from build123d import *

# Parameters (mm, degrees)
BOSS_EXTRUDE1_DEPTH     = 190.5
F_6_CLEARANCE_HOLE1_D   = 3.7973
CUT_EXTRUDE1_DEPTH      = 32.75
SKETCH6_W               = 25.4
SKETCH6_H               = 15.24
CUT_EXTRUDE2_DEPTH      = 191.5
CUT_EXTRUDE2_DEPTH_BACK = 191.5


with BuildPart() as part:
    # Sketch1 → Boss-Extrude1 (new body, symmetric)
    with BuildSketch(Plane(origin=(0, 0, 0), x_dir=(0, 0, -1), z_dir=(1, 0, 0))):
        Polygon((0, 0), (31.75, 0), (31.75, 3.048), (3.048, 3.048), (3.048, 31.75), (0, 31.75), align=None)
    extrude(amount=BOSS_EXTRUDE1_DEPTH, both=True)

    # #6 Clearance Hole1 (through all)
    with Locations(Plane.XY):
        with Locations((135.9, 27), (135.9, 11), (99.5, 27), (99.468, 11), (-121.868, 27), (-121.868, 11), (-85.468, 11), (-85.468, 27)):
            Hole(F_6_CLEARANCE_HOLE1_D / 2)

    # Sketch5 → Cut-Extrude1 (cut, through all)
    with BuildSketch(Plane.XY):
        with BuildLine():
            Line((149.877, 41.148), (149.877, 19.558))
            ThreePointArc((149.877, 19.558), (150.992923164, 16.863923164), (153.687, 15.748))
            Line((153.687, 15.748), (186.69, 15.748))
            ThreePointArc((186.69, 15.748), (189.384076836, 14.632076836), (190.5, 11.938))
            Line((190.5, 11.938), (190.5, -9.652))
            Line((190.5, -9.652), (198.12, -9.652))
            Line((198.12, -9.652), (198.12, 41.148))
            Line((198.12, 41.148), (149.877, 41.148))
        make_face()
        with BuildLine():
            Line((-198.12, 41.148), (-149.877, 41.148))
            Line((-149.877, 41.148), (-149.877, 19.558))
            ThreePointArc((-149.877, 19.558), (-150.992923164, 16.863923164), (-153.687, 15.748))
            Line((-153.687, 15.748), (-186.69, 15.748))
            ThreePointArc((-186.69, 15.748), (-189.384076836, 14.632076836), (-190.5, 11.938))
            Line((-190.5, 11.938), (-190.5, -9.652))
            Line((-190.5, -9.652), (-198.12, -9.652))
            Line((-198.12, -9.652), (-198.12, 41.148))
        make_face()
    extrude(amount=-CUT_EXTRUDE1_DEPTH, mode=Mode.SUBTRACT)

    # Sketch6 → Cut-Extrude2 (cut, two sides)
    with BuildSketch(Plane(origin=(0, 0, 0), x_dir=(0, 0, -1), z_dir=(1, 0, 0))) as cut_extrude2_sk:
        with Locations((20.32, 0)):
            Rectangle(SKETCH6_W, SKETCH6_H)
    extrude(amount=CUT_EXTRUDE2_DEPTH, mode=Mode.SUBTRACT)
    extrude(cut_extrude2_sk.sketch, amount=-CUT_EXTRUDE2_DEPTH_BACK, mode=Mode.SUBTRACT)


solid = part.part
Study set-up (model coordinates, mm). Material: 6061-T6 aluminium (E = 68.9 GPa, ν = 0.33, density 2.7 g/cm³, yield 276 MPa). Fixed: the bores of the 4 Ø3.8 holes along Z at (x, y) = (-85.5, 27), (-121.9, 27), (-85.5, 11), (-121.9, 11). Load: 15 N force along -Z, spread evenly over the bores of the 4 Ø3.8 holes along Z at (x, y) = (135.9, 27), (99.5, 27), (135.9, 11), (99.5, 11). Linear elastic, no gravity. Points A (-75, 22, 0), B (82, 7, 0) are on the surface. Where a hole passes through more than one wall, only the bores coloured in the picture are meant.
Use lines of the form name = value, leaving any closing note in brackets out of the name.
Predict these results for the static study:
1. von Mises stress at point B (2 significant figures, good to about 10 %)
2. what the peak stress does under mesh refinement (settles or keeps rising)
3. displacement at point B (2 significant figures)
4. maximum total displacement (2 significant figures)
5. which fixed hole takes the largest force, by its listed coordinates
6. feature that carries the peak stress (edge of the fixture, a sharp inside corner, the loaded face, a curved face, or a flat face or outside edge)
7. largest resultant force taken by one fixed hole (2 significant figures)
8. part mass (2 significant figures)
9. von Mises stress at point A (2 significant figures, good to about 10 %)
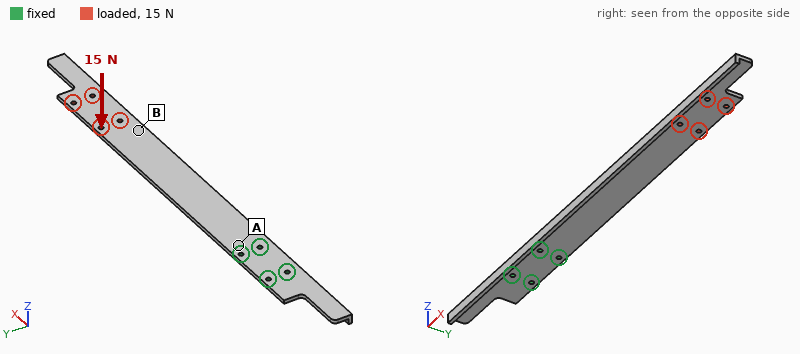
von Mises stress at point B = 6.0 MPa
what the peak stress does under mesh refinement = keeps rising
displacement at point B = 2.0 mm
maximum total displacement = 4.2 mm
which fixed hole takes the largest force, by its listed coordinates = (-85.5, 11)
feature that carries the peak stress = edge of the fixture
largest resultant force taken by one fixed hole = 190 N
part mass = 100 g
von Mises stress at point A = 23 MPa
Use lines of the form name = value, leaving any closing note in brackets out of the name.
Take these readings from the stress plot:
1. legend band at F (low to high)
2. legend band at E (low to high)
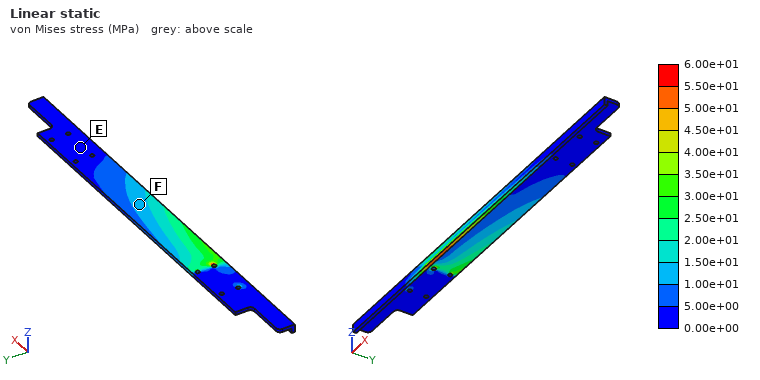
legend band at F = 1.00e+01 to 1.50e+01 MPa
legend band at E = 0.00e+00 to 5.00e+00 MPa
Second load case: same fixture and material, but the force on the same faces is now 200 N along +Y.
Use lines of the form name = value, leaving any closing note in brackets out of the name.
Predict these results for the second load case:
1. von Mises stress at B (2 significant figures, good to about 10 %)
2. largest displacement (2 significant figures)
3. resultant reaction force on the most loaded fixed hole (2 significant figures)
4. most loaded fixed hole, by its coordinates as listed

von Mises stress at B = 10 MPa
largest displacement = 3.6 mm
resultant reaction force on the most loaded fixed hole = 1.8 kN
most loaded fixed hole, by its coordinates as listed = (-85.5, 27)
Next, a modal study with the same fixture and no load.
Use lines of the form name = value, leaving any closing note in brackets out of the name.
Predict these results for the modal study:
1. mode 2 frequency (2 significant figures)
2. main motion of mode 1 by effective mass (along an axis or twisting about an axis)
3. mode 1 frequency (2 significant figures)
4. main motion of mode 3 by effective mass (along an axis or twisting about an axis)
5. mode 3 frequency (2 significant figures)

mode 2 frequency = 340 Hz
main motion of mode 1 by effective mass = along Z
mode 1 frequency = 59 Hz
main motion of mode 3 by effective mass = along Y
mode 3 frequency = 390 Hz
